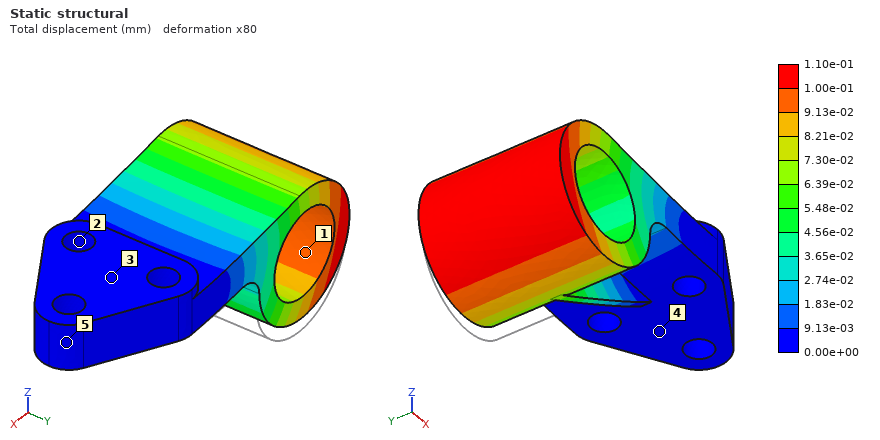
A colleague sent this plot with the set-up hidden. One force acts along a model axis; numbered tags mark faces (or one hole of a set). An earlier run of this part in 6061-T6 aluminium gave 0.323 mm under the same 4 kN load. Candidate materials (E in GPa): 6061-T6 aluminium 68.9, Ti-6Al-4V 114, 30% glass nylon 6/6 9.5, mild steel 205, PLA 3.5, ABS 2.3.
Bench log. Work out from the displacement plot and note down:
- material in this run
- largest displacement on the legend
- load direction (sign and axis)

mild steel
1.10e-01 mm
+Z
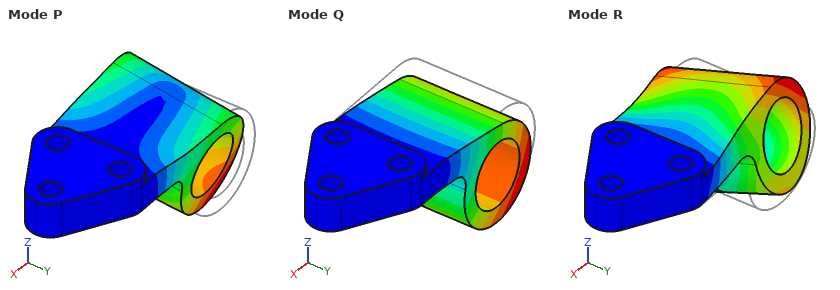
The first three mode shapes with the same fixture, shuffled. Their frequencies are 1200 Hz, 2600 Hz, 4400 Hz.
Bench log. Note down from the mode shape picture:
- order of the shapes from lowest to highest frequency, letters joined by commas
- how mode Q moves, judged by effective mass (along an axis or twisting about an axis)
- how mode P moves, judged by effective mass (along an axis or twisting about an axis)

Q, P, R
along Z
along Y
